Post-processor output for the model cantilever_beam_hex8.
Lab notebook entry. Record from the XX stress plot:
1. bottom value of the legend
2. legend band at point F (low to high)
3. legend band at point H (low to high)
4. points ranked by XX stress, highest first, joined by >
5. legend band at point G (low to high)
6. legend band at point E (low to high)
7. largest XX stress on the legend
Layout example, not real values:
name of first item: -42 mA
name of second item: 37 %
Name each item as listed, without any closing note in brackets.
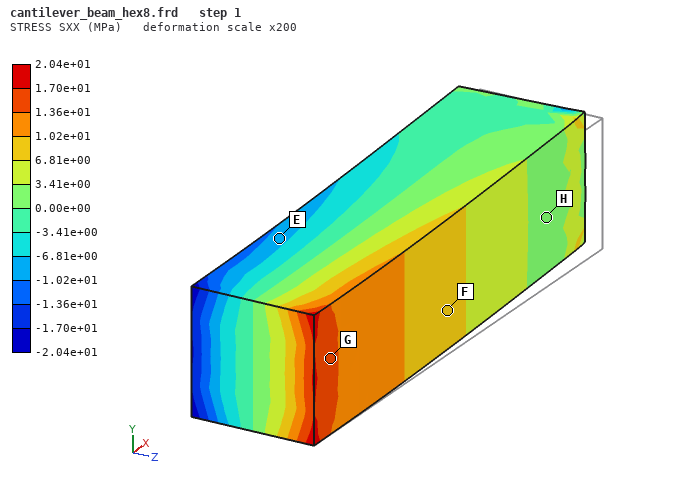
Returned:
bottom value of the legend: -2.04e+01 MPa
legend band at point F: 6.81e+00 to 1.02e+01 MPa
legend band at point H: 0.00e+00 to 3.41e+00 MPa
points ranked by XX stress, highest first, joined by >: G > F > H > E
legend band at point G: 1.36e+01 to 1.70e+01 MPa
legend band at point E: -1.02e+01 to -6.81e+00 MPa
largest XX stress on the legend: 2.04e+01 MPa
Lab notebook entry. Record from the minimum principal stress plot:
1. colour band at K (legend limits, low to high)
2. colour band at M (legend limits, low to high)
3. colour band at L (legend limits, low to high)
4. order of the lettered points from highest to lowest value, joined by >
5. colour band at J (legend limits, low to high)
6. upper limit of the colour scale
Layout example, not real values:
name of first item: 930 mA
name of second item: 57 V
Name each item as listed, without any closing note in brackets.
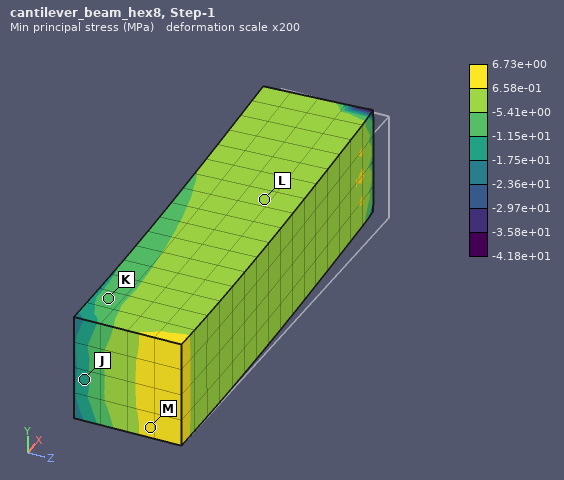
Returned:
colour band at K: -1.15e+01 to -5.41e+00 MPa
colour band at M: 6.58e-01 to 6.73e+00 MPa
colour band at L: -5.41e+00 to 6.58e-01 MPa
order of the lettered points from highest to lowest value, joined by >: M > L > K > J
colour band at J: -1.75e+01 to -1.15e+01 MPa
upper limit of the colour scale: 6.73e+00 MPa
